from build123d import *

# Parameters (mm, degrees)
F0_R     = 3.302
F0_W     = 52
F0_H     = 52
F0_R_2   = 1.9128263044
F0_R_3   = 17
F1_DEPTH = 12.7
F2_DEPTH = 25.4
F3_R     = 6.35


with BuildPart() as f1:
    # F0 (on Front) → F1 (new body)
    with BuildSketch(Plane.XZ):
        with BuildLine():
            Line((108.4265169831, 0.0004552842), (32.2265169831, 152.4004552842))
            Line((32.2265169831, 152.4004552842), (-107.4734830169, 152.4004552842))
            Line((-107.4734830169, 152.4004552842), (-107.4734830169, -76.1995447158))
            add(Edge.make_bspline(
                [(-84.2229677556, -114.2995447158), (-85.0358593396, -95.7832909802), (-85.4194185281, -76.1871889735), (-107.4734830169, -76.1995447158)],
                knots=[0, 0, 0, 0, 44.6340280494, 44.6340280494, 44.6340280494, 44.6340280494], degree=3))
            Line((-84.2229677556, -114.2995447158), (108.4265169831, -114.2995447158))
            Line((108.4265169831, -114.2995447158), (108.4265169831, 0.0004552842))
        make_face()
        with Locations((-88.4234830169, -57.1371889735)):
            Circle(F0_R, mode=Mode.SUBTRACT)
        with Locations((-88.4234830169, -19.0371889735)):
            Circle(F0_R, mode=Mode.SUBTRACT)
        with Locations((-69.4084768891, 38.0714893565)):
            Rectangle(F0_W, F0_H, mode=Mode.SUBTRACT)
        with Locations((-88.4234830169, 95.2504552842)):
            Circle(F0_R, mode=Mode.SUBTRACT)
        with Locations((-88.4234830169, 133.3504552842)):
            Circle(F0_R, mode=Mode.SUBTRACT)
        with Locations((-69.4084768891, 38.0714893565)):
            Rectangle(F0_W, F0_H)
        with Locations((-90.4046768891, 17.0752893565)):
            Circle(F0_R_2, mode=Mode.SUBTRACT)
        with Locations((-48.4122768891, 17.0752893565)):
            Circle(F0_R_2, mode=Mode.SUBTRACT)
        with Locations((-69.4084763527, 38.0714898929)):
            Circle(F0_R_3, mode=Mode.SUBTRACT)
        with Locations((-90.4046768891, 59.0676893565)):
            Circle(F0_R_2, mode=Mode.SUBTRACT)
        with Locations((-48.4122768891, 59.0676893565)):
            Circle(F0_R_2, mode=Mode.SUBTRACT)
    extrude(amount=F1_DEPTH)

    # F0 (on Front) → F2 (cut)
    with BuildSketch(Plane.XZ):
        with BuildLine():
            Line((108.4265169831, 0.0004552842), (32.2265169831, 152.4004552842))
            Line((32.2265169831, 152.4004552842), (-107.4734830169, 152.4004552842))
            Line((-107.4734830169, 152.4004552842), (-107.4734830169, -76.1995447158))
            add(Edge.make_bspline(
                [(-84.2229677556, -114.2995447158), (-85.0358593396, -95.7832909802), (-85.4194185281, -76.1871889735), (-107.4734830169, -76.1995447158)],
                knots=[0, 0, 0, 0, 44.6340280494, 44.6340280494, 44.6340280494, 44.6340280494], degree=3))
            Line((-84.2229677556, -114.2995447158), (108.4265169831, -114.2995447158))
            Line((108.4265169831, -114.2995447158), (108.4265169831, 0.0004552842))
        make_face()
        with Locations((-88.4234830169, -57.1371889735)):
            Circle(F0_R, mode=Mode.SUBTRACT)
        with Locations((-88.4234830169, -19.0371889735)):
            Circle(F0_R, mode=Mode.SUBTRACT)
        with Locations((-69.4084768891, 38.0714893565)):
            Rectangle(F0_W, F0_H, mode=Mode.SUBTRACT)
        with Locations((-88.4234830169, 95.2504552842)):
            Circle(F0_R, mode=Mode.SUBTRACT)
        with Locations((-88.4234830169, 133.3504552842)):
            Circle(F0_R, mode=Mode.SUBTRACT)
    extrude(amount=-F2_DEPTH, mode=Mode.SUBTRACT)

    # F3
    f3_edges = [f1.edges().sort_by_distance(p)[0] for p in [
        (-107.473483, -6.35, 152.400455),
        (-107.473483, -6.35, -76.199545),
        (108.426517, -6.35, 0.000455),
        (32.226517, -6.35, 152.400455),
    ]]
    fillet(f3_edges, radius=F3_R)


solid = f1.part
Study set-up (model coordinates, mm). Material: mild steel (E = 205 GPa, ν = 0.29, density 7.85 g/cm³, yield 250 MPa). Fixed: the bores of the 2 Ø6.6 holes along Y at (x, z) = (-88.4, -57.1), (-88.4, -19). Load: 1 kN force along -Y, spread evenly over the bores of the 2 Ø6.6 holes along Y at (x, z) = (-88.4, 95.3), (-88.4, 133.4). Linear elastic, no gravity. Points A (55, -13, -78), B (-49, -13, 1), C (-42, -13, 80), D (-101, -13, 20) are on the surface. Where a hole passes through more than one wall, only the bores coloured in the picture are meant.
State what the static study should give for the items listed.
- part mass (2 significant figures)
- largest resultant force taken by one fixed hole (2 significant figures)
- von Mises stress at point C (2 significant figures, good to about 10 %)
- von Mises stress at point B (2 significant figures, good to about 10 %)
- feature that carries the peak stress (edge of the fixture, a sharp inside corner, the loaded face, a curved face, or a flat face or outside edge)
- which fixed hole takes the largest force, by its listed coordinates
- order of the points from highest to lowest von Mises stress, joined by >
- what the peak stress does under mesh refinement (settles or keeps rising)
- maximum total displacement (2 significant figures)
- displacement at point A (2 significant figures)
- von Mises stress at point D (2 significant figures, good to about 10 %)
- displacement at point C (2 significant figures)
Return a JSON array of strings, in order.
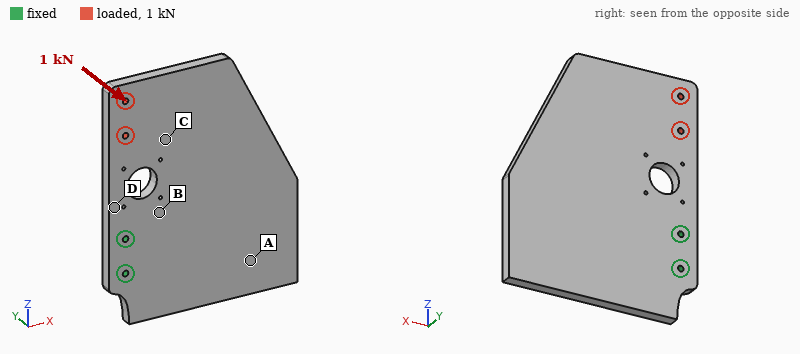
["5.0 kg", "2.9 kN", "16 MPa", "25 MPa", "edge of the fixture", "(-88.4, -19)", "D > B > C > A", "keeps rising", "0.37 mm", "0.060 mm", "45 MPa", "0.16 mm"]
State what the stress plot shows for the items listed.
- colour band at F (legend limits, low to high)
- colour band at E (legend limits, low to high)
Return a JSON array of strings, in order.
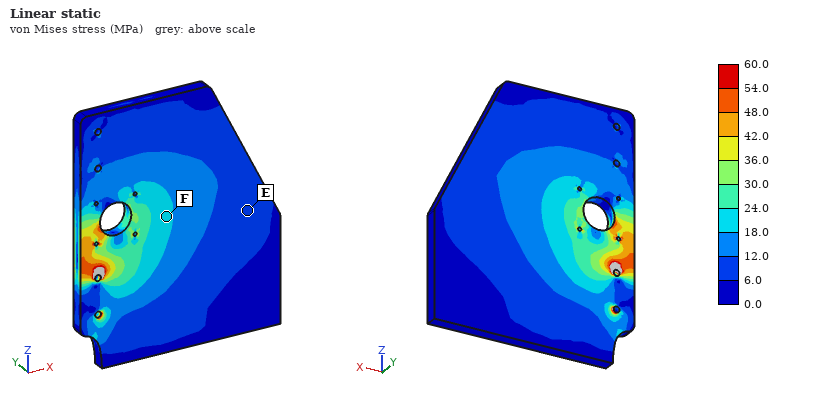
["18.0 to 24.0 MPa", "6.0 to 12.0 MPa"]
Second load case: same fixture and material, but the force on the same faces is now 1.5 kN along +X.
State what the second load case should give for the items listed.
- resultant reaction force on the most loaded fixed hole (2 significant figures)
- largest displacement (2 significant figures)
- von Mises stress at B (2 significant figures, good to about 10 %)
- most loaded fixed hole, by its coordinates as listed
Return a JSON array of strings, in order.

["6.1 kN", "29 µm", "4.1 MPa", "(-88.4, -19)"]
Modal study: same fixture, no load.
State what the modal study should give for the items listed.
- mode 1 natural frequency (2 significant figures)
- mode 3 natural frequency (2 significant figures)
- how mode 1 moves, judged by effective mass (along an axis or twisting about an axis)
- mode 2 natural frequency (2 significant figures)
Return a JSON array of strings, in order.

["200 Hz", "730 Hz", "along Y", "280 Hz"]
